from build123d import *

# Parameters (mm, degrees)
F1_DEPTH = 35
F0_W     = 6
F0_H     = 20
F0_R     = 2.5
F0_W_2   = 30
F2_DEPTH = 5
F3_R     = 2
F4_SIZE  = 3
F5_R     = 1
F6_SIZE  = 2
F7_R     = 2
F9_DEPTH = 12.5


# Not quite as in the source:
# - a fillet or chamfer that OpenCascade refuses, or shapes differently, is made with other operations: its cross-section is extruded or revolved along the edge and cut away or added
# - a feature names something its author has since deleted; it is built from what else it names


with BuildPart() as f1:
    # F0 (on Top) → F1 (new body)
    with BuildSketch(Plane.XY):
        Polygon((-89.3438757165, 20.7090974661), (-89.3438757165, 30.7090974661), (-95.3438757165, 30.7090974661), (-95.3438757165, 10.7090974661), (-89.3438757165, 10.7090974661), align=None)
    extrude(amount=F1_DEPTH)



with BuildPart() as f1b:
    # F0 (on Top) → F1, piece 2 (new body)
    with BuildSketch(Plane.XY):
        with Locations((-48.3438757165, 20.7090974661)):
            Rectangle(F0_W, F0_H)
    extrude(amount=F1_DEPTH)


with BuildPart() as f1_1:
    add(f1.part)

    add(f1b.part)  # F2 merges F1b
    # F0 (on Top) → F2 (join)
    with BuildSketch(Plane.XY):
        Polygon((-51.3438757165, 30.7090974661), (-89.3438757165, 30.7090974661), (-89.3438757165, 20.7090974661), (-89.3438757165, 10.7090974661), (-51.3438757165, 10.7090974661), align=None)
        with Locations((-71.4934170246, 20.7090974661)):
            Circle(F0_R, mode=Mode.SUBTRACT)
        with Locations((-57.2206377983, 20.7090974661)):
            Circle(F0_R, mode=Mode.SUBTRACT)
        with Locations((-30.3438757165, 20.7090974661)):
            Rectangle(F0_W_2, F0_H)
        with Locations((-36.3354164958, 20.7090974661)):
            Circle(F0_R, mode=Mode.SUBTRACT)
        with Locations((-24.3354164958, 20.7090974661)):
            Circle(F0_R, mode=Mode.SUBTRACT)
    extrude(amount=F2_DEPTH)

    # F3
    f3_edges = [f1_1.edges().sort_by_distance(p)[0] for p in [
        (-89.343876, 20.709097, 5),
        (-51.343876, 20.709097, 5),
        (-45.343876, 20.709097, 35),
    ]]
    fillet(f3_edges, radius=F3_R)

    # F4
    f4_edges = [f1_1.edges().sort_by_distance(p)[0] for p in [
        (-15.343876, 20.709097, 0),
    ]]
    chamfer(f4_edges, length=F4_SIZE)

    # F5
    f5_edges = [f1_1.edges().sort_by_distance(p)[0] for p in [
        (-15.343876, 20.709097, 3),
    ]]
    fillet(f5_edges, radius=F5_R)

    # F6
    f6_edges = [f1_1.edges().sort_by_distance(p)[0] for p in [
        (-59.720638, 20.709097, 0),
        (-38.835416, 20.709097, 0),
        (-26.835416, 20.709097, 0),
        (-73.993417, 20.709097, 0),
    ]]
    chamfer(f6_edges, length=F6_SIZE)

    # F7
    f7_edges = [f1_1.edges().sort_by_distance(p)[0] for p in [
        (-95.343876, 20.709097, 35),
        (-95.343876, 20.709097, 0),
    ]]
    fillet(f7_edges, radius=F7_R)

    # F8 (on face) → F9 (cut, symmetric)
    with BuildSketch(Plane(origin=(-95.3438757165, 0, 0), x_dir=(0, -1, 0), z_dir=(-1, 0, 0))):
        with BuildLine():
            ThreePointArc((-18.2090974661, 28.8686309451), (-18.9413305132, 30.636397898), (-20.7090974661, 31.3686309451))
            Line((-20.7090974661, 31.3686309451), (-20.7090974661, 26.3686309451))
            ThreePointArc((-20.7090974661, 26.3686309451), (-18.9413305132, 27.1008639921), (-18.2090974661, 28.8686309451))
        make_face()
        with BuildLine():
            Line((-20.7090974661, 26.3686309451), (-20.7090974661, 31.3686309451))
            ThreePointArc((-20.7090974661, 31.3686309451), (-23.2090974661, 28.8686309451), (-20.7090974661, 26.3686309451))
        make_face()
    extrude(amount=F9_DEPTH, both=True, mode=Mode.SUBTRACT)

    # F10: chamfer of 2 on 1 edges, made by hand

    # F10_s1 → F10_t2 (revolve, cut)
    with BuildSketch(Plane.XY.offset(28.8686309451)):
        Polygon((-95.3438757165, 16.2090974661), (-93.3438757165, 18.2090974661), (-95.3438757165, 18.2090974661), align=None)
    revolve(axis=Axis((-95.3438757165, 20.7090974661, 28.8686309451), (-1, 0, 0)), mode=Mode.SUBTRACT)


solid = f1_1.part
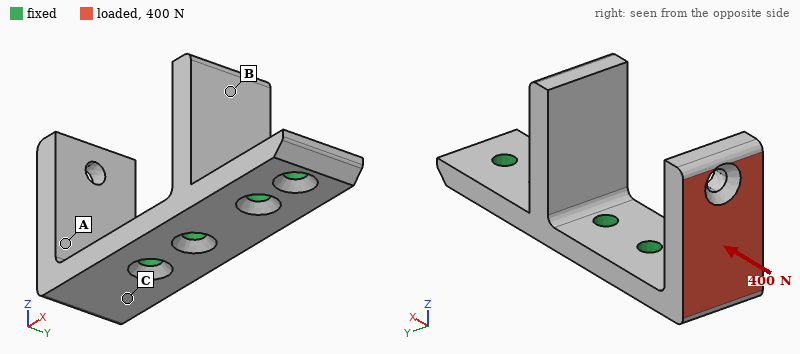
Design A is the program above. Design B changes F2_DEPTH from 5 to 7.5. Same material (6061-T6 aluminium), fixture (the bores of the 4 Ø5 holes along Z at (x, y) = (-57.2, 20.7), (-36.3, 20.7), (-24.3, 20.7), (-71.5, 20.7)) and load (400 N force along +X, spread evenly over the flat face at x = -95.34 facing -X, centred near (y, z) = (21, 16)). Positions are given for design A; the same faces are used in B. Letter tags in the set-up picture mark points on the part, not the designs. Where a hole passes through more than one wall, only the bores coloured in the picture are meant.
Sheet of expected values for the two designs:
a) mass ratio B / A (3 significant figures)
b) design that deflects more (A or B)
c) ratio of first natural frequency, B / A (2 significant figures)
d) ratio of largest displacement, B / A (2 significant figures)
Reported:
1.22
A
1.8
0.33
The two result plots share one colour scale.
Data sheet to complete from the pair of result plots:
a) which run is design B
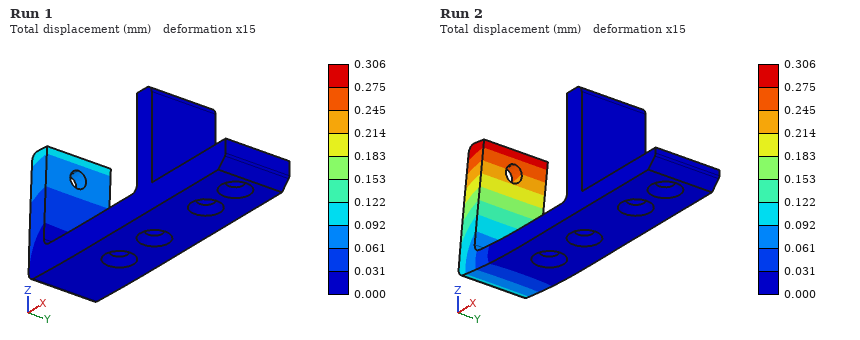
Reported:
Run 1
